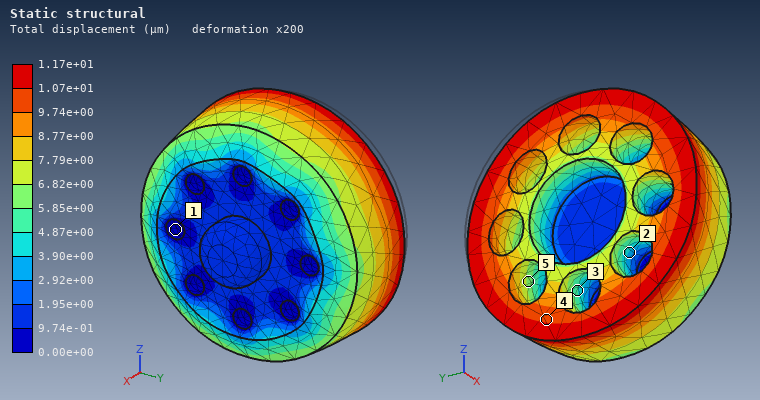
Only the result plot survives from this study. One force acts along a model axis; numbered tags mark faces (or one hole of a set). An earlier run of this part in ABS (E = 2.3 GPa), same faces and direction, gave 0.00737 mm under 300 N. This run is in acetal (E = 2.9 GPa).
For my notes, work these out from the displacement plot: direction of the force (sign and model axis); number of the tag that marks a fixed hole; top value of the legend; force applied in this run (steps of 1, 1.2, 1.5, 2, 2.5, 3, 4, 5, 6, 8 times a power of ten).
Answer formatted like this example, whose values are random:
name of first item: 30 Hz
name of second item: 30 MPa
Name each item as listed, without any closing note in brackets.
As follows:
direction of the force: +X
number of the tag that marks a fixed hole: 1
top value of the legend: 1.17e+01 µm
force applied in this run: 600 N
